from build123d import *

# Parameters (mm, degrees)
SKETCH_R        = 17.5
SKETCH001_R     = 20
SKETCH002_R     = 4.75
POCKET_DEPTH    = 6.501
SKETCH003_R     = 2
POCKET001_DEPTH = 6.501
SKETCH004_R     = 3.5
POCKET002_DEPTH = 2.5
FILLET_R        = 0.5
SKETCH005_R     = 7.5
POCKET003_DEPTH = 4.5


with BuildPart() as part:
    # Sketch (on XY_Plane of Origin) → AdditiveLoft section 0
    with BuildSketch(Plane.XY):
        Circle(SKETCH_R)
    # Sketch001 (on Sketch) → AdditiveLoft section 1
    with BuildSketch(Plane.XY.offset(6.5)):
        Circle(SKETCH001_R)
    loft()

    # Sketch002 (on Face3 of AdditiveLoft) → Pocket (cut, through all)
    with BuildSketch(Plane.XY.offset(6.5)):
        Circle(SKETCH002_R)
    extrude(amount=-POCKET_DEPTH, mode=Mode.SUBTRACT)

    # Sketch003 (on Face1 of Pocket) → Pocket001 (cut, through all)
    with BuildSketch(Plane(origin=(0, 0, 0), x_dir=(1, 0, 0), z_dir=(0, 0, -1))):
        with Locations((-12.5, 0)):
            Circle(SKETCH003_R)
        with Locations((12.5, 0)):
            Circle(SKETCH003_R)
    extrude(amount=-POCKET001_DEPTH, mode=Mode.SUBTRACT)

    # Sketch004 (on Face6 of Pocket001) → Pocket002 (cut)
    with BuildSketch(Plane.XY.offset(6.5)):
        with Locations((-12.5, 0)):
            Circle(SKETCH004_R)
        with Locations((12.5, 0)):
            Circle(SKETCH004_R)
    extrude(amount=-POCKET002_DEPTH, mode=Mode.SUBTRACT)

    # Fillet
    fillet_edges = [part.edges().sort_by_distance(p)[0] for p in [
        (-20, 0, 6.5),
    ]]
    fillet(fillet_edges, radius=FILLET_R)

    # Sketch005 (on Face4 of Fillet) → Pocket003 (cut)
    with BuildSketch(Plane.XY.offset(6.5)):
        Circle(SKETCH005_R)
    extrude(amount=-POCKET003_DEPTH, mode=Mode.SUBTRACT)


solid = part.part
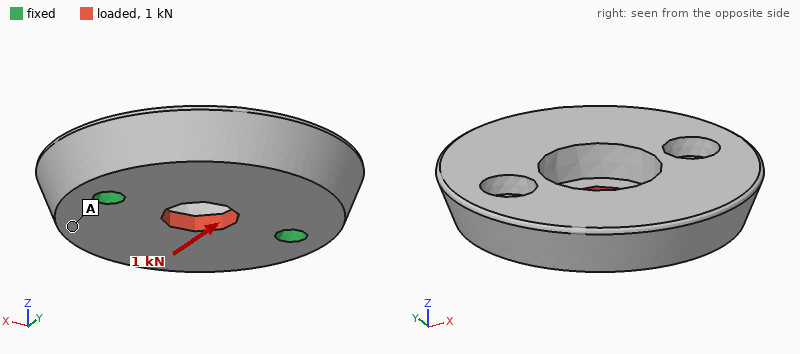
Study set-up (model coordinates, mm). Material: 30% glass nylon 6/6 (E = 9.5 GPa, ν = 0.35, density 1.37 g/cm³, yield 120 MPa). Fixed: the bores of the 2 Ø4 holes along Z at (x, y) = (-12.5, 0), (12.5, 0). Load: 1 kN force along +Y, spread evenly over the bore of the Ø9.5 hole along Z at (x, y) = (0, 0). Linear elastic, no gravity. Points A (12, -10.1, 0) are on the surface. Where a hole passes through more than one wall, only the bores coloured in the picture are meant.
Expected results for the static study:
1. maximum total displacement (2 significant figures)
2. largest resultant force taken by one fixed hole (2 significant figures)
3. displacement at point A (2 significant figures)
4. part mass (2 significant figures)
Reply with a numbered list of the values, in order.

1. 33 µm
2. 500 N
3. 15 µm
4. 8.1 g
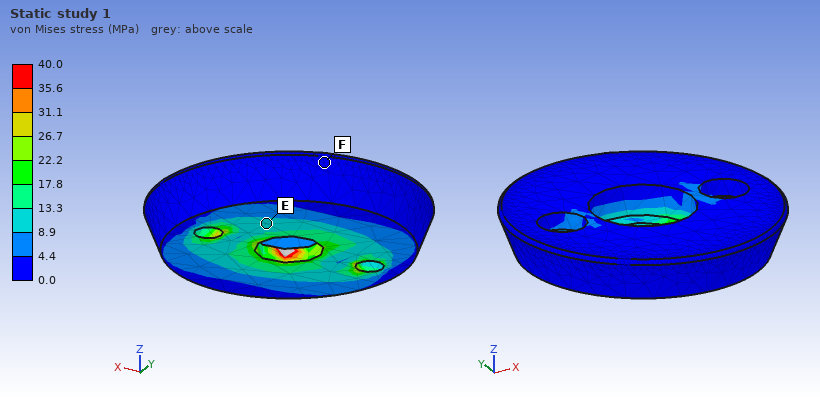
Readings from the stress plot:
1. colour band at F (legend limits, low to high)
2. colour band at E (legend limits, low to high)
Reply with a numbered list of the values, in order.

1. 0.0 to 4.4 MPa
2. 8.9 to 13.3 MPa
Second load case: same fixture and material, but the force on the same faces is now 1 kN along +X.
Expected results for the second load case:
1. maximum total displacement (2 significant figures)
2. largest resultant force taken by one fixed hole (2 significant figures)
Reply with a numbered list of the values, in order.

1. 18 µm
2. 500 N
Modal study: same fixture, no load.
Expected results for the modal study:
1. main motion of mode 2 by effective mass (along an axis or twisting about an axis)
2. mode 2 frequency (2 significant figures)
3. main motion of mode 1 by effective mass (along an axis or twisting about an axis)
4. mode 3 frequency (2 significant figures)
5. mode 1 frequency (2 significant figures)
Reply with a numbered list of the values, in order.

1. along Z
2. 6600 Hz
3. twisting about X
4. 13 kHz
5. 5000 Hz
